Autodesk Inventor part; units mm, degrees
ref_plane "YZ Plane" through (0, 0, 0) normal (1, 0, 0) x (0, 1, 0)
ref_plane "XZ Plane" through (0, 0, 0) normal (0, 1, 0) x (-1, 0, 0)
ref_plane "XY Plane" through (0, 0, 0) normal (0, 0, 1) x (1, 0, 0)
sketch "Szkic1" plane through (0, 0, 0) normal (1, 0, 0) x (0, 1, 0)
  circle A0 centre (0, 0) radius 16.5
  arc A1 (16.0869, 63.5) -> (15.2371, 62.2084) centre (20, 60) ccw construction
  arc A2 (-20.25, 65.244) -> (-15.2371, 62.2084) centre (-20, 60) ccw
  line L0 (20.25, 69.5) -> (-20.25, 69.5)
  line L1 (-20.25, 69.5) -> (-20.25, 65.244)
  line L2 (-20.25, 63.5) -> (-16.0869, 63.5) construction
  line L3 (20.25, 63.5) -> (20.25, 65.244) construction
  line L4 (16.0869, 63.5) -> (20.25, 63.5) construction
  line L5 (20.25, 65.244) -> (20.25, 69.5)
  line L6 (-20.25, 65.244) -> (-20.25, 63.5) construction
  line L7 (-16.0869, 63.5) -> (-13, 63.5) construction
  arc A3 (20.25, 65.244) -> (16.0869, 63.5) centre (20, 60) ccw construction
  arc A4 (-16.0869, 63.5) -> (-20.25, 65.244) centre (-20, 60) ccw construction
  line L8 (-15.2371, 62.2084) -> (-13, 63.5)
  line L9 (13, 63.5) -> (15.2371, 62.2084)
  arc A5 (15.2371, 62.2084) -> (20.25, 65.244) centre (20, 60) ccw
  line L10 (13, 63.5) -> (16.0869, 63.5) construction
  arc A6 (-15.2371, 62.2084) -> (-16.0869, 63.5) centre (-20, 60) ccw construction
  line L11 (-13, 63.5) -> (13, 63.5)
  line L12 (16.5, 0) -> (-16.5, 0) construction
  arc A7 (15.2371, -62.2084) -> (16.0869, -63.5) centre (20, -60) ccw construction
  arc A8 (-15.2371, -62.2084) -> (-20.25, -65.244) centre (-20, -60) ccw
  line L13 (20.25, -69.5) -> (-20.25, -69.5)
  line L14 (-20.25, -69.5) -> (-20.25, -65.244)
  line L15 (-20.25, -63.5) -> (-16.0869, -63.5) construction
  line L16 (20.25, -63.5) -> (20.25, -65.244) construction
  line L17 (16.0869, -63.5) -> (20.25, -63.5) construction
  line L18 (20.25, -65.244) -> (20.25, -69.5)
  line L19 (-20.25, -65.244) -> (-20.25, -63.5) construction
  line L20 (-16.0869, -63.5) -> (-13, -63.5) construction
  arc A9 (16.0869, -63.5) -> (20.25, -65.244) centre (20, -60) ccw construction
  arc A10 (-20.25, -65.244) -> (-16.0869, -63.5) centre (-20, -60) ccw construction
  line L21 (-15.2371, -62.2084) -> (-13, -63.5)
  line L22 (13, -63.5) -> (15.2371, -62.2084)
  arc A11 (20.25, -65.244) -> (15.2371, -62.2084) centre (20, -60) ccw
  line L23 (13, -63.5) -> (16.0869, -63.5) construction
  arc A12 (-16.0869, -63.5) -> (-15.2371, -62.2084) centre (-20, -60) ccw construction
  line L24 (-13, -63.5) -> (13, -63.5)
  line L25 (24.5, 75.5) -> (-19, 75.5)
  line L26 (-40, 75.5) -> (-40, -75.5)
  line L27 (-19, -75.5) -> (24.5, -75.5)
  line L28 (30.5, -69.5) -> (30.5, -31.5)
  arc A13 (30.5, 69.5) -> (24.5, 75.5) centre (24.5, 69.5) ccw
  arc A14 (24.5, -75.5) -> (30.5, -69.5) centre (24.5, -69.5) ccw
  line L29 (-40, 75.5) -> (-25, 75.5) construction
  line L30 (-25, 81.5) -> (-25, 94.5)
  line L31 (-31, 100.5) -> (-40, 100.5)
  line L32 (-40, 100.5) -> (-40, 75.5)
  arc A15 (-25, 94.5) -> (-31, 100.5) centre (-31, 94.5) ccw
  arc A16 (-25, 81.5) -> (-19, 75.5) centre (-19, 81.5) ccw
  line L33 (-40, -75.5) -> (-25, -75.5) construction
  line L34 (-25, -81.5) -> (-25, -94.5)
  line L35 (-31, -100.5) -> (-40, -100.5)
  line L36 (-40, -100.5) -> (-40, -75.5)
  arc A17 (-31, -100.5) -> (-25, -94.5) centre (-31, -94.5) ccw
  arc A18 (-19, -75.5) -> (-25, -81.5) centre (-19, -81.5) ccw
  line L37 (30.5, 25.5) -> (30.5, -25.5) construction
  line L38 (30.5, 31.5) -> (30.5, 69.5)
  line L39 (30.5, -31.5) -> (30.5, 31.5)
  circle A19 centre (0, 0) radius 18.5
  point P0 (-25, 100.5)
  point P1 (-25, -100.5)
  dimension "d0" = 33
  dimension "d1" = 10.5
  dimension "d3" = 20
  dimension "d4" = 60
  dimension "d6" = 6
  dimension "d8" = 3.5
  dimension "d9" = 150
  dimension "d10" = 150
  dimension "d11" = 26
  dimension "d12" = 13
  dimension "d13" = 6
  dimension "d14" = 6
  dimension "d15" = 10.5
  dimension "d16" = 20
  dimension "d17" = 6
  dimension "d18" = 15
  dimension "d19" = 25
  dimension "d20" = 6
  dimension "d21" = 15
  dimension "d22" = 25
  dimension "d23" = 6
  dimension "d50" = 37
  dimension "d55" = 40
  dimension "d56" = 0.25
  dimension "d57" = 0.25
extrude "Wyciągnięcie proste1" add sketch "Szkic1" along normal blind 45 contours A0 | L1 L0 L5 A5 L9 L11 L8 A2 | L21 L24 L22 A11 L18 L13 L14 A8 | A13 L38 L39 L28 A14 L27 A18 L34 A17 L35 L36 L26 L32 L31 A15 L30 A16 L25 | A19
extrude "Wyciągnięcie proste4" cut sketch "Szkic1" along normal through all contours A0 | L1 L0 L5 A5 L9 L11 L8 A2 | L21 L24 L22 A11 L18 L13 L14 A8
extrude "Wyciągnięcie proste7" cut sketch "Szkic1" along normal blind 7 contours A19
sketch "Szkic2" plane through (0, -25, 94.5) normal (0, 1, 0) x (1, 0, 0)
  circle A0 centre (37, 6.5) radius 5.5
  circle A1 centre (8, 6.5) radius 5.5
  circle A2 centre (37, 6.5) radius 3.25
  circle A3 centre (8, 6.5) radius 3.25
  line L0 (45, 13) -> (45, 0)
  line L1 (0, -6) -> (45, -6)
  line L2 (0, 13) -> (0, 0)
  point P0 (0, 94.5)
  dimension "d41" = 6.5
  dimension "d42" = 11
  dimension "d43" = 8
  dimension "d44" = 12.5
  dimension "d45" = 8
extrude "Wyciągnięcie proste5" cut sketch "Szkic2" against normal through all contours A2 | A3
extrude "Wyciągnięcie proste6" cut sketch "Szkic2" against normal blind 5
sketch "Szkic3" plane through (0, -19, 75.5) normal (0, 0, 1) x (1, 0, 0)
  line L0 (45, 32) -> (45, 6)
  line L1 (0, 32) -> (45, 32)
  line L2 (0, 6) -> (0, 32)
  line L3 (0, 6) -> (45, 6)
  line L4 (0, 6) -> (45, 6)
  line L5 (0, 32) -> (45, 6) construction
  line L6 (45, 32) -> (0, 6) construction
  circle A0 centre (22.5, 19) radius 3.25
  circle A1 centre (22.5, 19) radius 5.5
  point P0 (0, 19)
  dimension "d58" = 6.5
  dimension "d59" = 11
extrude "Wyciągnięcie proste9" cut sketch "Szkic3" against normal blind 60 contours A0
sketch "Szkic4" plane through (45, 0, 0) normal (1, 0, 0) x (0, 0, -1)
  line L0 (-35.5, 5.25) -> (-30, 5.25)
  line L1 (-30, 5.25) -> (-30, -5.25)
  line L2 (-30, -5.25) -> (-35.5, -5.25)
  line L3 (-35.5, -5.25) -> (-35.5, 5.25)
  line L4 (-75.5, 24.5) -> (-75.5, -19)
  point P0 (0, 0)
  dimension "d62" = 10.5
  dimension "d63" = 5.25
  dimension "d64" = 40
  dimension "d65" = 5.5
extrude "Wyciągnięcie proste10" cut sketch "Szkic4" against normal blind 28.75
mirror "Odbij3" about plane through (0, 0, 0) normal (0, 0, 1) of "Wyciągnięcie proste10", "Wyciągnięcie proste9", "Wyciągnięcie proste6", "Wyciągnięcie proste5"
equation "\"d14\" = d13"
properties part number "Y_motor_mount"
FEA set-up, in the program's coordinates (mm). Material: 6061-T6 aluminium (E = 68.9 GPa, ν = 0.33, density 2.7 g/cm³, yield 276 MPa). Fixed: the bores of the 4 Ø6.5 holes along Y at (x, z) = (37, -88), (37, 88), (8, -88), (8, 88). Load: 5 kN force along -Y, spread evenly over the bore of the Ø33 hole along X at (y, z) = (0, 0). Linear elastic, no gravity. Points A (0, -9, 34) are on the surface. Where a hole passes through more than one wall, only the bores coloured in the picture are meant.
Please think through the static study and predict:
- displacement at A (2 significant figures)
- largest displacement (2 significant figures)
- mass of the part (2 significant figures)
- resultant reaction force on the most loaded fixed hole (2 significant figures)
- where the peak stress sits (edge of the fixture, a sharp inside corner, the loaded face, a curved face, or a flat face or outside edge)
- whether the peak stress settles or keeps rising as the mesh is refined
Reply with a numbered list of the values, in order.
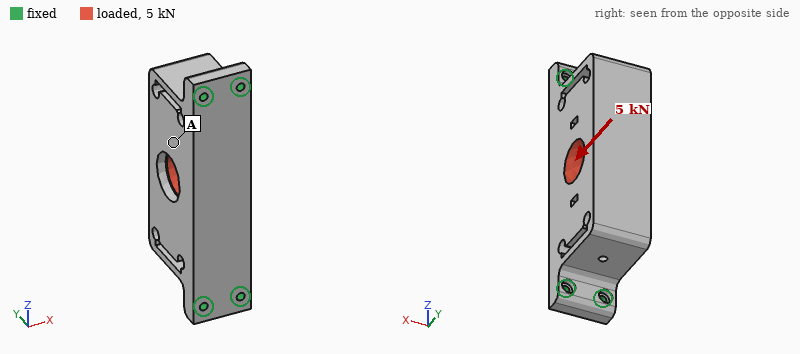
1. 19 µm
2. 28 µm
3. 1.1 kg
4. 1.9 kN
5. edge of the fixture
6. keeps rising
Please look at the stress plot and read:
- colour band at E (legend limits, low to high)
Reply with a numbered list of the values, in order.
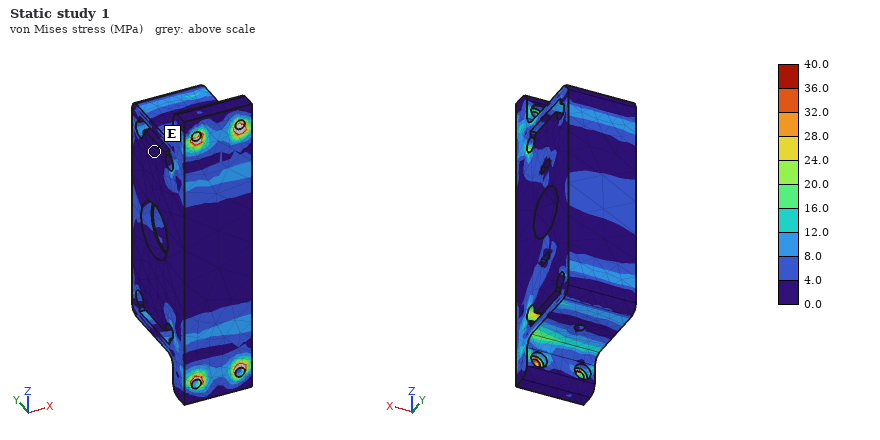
1. 0.0 to 4.0 MPa
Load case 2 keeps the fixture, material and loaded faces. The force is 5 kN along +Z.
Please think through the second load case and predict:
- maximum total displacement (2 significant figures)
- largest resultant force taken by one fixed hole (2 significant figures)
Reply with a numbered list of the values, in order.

1. 10 µm
2. 1.4 kN
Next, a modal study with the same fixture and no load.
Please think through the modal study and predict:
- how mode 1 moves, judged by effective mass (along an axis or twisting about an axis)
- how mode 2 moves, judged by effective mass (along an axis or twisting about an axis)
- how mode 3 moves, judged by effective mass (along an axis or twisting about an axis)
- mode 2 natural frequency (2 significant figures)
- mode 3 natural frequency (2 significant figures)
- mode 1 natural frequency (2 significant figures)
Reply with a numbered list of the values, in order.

1. along X
2. along Y
3. along Z
4. 2500 Hz
5. 3700 Hz
6. 1600 Hz
